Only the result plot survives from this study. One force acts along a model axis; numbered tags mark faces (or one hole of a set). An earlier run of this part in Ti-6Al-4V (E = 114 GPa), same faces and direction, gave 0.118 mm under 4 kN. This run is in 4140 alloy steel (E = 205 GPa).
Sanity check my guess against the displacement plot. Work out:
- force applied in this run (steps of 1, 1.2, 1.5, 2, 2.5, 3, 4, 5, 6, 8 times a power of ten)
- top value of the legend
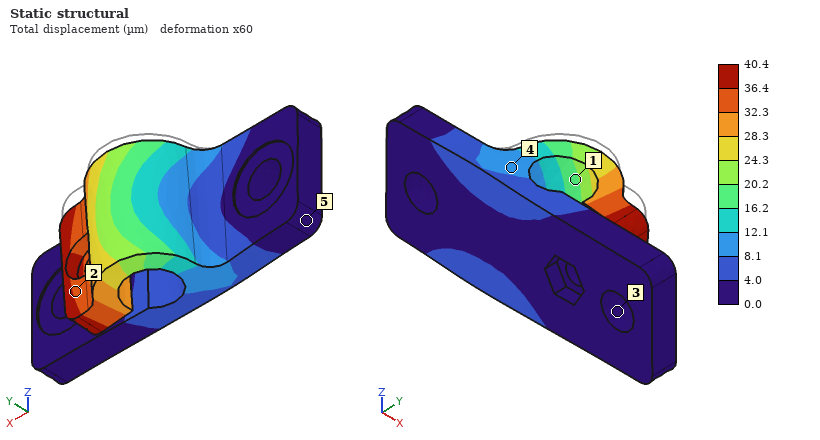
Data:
2.5 kN
40.4 µm
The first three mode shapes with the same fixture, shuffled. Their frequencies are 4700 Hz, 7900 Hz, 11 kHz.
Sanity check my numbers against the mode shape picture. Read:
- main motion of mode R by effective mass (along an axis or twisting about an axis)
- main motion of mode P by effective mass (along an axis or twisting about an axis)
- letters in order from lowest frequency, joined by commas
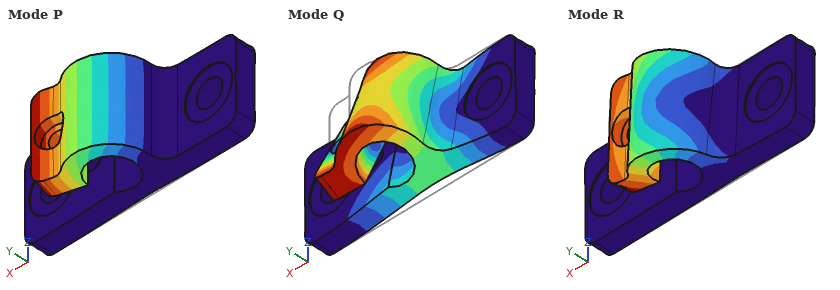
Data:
along Z
along Y
P, R, Q
